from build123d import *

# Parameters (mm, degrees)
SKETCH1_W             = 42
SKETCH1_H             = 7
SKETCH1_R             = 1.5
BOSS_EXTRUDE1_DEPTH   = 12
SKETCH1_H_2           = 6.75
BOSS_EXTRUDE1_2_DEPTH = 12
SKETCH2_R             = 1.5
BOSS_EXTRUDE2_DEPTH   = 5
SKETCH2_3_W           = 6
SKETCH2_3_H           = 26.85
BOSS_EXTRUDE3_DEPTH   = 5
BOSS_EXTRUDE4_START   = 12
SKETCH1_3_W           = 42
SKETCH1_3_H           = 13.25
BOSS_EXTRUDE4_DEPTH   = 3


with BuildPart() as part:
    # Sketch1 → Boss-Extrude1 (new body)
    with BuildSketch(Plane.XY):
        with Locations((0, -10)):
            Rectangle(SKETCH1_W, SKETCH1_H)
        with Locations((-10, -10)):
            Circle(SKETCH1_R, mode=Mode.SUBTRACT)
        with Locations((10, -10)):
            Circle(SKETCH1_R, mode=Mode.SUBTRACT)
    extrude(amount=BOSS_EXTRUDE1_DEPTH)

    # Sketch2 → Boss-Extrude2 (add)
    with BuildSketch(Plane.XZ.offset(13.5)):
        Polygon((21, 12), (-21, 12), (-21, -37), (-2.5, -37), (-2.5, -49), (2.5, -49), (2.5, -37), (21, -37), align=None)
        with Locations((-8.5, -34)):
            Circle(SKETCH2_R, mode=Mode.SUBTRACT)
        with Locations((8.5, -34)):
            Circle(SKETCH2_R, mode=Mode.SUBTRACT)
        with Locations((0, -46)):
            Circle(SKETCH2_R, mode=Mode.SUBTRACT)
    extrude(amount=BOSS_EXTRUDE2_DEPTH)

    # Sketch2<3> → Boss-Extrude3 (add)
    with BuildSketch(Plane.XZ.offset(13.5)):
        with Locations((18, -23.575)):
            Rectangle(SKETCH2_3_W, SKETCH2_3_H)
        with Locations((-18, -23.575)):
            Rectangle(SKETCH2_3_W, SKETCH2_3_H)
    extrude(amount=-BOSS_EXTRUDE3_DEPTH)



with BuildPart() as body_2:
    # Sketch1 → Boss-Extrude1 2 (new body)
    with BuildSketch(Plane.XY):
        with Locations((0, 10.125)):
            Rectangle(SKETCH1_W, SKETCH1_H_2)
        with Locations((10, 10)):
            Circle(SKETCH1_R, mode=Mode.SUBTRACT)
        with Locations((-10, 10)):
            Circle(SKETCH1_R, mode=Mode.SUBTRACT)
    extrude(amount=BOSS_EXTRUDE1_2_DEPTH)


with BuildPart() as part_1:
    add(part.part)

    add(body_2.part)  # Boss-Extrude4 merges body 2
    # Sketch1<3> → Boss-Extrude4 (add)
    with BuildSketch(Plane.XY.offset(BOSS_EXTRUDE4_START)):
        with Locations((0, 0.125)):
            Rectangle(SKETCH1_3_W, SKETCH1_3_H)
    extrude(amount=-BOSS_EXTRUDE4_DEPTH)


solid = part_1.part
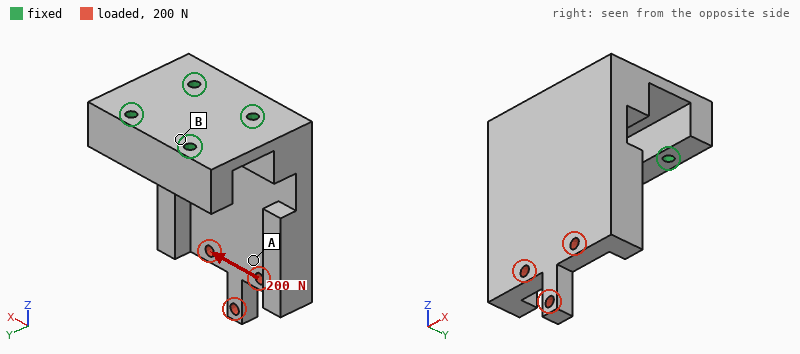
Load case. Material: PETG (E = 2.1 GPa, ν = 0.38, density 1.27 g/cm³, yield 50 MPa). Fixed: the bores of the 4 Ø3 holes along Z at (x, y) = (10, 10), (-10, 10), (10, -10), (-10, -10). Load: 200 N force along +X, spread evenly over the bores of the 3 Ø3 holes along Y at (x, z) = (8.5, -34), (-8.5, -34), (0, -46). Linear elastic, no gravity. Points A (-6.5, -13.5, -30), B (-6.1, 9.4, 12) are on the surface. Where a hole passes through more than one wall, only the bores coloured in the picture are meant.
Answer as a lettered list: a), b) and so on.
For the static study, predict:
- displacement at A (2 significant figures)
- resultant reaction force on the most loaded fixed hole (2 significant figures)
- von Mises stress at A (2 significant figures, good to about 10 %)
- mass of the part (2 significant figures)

a) 0.18 mm
b) 320 N
c) 4.0 MPa
d) 26 g
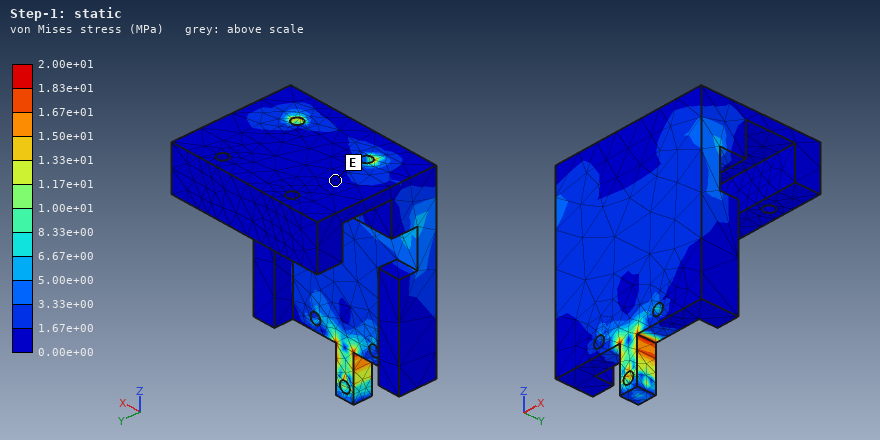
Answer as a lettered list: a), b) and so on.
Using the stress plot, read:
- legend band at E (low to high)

a) 0.00e+00 to 1.67e+00 MPa
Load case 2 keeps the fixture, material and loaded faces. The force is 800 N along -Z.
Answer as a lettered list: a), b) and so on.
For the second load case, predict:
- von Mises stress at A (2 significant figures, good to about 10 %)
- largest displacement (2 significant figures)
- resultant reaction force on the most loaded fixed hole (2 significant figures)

a) 6.0 MPa
b) 0.37 mm
c) 410 N
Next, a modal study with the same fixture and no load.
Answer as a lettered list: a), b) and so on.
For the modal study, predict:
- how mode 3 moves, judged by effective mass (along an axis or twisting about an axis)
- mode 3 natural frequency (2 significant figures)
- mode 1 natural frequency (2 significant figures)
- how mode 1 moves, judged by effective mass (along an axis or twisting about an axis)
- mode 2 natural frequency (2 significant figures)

a) along X
b) 2100 Hz
c) 570 Hz
d) along Y
e) 1200 Hz
